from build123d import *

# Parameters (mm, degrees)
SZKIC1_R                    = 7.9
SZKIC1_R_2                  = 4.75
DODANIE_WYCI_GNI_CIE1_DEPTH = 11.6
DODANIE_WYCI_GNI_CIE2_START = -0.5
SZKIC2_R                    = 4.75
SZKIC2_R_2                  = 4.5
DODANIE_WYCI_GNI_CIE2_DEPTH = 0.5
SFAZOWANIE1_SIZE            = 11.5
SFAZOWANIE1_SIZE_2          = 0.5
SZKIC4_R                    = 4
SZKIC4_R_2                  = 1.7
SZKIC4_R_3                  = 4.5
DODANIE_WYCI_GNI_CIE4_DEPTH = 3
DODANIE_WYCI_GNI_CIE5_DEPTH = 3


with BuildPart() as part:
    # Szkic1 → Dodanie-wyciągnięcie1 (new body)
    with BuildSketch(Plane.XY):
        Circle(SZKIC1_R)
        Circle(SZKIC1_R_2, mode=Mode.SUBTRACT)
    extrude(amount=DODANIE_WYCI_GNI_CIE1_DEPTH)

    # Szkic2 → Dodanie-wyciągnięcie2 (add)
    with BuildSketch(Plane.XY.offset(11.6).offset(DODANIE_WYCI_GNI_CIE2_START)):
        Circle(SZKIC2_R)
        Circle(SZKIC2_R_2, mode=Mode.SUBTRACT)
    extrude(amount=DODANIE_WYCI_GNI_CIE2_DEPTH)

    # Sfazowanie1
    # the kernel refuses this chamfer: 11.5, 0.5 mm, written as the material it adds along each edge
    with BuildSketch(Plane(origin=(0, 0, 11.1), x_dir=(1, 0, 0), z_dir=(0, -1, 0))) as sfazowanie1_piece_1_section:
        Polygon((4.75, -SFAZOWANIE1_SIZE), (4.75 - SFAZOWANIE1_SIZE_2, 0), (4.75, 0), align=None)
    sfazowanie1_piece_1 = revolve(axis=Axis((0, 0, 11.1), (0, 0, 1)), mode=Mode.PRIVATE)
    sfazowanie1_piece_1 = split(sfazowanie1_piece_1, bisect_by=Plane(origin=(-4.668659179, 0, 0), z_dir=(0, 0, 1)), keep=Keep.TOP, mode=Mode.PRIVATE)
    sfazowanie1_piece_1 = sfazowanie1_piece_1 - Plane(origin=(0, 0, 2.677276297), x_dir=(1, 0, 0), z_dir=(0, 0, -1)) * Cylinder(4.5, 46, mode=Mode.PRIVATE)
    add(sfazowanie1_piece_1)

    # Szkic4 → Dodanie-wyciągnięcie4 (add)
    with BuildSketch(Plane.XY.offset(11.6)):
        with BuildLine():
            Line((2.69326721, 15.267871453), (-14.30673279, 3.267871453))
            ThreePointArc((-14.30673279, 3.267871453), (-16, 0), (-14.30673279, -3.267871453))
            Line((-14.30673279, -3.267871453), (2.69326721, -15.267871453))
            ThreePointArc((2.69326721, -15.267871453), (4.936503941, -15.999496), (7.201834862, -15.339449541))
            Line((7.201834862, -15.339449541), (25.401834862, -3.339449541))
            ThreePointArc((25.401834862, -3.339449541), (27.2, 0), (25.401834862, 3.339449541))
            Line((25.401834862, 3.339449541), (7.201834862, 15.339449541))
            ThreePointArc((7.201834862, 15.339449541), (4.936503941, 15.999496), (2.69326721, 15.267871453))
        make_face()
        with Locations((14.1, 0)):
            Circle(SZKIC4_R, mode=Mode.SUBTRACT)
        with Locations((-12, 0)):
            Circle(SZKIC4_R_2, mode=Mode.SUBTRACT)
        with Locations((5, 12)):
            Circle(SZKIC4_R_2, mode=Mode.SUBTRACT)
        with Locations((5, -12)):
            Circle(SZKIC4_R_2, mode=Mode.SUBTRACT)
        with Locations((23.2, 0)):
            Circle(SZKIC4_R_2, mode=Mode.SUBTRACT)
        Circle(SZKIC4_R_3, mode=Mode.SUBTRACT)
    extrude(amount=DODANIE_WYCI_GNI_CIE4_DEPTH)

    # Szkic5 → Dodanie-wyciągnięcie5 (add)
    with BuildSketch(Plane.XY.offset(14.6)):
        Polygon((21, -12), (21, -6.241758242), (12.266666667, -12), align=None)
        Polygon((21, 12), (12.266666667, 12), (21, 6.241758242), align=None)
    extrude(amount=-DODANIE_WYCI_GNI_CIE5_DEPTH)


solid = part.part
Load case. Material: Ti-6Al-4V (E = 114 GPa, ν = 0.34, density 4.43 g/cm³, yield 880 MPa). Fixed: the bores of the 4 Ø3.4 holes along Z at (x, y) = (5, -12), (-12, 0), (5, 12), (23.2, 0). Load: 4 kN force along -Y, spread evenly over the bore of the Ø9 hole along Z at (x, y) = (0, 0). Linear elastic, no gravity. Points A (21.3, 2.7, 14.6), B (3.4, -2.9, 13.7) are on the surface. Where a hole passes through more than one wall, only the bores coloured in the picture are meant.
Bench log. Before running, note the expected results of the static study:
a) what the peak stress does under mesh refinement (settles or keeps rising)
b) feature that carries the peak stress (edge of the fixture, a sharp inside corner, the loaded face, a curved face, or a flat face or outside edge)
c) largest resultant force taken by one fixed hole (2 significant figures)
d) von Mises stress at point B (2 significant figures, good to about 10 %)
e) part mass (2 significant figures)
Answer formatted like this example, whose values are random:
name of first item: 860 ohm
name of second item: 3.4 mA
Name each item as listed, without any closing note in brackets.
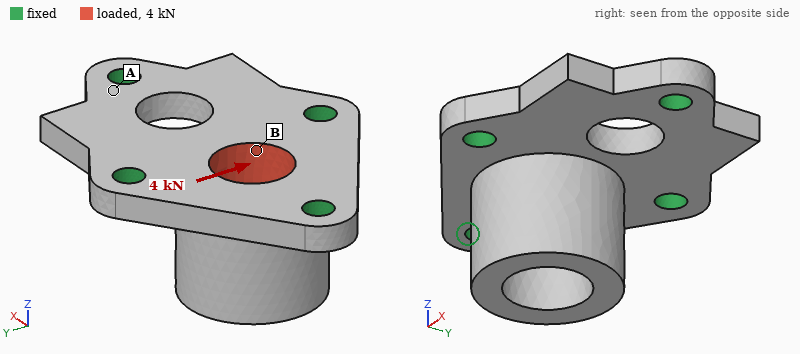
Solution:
what the peak stress does under mesh refinement: keeps rising
feature that carries the peak stress: edge of the fixture
largest resultant force taken by one fixed hole: 1.6 kN
von Mises stress at point B: 37 MPa
part mass: 16 g
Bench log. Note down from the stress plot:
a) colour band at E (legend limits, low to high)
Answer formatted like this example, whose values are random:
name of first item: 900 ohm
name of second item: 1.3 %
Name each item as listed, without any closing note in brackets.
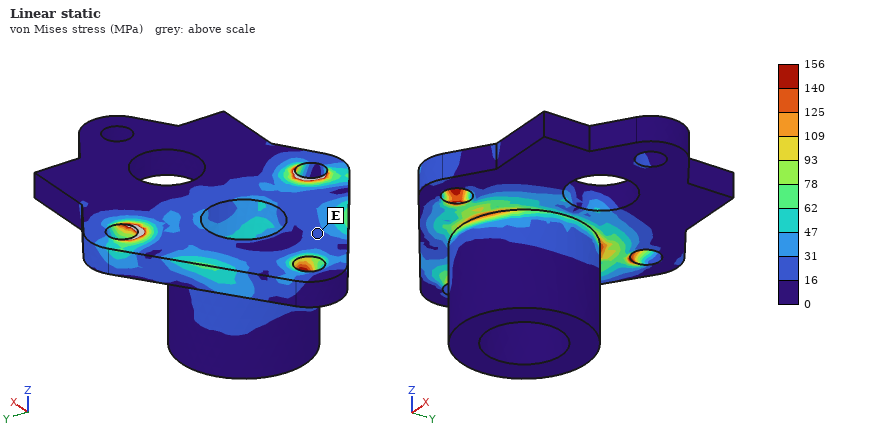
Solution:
colour band at E: 16 to 31 MPa
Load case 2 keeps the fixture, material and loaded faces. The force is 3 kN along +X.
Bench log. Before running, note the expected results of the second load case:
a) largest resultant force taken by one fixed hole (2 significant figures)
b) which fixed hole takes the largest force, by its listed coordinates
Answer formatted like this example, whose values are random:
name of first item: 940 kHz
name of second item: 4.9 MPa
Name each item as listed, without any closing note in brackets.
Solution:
largest resultant force taken by one fixed hole: 1.4 kN
which fixed hole takes the largest force, by its listed coordinates: (-12, 0)
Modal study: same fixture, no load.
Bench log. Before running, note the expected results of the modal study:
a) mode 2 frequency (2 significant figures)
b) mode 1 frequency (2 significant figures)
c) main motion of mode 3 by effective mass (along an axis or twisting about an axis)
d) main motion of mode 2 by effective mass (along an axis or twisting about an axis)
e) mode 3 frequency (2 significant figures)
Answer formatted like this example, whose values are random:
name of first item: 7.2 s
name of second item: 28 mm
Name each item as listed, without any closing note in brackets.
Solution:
mode 2 frequency: 21 kHz
mode 1 frequency: 20 kHz
main motion of mode 3 by effective mass: along Z
main motion of mode 2 by effective mass: along Y
mode 3 frequency: 27 kHz
